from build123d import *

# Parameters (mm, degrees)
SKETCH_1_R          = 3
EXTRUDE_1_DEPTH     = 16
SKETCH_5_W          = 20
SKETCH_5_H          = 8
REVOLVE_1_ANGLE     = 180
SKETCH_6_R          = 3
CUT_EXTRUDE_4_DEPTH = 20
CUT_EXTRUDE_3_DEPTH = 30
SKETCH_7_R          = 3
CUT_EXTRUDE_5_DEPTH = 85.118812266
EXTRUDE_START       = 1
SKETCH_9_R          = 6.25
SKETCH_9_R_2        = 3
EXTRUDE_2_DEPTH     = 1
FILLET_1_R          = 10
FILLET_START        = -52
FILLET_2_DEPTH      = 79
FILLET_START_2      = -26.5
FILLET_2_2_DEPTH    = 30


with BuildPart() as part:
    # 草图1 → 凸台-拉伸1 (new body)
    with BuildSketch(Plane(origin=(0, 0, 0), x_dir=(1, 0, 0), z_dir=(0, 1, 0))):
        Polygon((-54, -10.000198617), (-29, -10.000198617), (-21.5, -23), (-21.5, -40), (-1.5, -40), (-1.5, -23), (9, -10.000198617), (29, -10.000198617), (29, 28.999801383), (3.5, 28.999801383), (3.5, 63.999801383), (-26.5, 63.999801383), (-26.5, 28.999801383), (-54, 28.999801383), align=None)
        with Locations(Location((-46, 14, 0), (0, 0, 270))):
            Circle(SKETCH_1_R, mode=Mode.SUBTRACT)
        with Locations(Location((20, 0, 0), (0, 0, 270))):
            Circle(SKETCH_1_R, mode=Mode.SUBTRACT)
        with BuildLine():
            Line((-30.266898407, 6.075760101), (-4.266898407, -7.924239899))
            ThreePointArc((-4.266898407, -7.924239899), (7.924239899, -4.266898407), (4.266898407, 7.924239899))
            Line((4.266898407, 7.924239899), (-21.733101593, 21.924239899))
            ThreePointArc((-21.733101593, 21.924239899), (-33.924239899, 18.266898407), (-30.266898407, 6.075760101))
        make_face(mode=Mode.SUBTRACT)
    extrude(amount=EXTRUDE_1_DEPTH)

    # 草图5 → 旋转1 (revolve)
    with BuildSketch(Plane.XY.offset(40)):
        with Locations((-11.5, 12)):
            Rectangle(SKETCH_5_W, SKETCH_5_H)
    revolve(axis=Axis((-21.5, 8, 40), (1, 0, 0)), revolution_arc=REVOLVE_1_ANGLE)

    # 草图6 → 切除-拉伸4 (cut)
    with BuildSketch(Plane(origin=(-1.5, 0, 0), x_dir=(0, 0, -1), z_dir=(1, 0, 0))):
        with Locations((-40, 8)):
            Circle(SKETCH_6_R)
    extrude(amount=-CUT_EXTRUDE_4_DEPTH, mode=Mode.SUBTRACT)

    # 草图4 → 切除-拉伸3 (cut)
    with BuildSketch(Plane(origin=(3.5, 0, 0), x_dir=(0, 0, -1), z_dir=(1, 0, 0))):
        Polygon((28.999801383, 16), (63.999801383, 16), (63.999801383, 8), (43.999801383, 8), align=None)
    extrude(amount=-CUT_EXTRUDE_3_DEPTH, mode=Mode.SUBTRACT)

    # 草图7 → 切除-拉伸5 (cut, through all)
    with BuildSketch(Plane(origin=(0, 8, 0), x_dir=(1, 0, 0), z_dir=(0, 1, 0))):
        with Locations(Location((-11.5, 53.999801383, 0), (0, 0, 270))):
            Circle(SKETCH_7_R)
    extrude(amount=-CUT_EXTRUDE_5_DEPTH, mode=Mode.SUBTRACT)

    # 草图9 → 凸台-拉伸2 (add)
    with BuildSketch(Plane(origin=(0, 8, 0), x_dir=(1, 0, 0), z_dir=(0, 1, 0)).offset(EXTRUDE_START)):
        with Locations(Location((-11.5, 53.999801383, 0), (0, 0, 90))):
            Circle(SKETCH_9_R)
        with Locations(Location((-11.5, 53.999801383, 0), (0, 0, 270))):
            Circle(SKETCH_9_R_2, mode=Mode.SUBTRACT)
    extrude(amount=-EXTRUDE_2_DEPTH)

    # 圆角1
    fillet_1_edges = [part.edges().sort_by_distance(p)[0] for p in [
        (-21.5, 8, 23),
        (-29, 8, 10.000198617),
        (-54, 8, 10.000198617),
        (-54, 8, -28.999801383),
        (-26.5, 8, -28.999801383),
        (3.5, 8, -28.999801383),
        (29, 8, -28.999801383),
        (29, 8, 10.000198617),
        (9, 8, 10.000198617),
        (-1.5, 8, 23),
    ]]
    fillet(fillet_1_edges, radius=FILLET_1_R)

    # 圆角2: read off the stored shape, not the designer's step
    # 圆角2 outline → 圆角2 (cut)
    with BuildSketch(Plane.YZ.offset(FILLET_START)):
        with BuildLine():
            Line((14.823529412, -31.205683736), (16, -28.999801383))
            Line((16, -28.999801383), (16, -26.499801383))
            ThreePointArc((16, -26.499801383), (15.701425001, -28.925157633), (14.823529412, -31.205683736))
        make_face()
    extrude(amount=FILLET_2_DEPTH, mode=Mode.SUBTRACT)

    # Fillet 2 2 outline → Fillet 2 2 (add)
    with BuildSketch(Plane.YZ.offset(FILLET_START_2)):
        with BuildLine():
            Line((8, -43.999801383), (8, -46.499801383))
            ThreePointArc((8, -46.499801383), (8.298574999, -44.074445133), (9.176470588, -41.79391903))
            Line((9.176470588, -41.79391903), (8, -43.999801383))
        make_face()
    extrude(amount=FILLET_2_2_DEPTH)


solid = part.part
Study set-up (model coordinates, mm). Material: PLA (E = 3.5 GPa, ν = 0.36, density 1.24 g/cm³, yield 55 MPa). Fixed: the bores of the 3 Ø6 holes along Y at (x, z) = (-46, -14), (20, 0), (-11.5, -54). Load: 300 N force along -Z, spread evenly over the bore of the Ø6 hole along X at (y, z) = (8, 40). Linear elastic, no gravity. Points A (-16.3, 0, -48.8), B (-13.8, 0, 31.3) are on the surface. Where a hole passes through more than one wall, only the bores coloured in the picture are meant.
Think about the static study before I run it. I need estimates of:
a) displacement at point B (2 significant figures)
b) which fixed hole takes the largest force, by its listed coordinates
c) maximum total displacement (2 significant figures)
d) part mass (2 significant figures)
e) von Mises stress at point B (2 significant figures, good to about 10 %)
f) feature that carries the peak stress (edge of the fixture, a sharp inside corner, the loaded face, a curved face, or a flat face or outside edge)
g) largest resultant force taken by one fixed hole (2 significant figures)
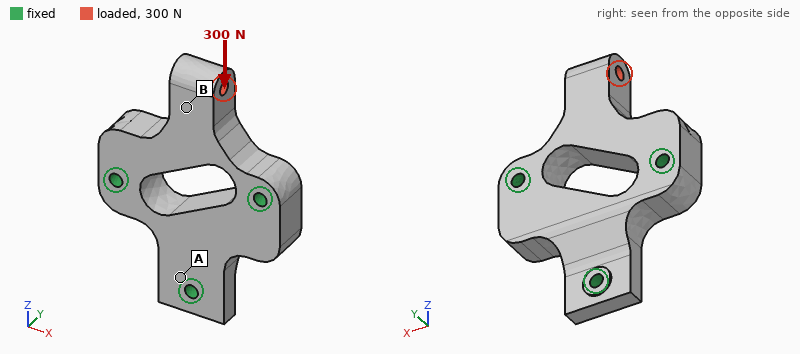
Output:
22 µm
(-46, -14)
28 µm
75 g
0.93 MPa
a curved face
200 N
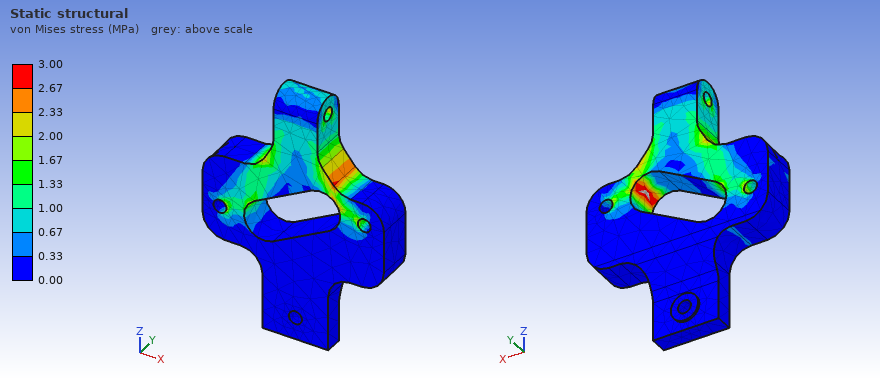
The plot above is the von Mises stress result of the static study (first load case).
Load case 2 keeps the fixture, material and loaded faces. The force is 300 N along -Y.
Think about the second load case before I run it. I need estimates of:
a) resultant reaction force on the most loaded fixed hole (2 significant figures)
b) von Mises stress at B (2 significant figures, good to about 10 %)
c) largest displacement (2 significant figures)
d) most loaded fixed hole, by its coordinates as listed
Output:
230 N
3.2 MPa
0.85 mm
(20, 0)
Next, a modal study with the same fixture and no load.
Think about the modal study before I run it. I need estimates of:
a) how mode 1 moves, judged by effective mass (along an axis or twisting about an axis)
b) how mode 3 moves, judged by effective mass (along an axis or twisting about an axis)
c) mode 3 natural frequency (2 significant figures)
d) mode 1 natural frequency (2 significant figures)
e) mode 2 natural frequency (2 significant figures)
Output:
along Y
along Y
4100 Hz
1200 Hz
3500 Hz
